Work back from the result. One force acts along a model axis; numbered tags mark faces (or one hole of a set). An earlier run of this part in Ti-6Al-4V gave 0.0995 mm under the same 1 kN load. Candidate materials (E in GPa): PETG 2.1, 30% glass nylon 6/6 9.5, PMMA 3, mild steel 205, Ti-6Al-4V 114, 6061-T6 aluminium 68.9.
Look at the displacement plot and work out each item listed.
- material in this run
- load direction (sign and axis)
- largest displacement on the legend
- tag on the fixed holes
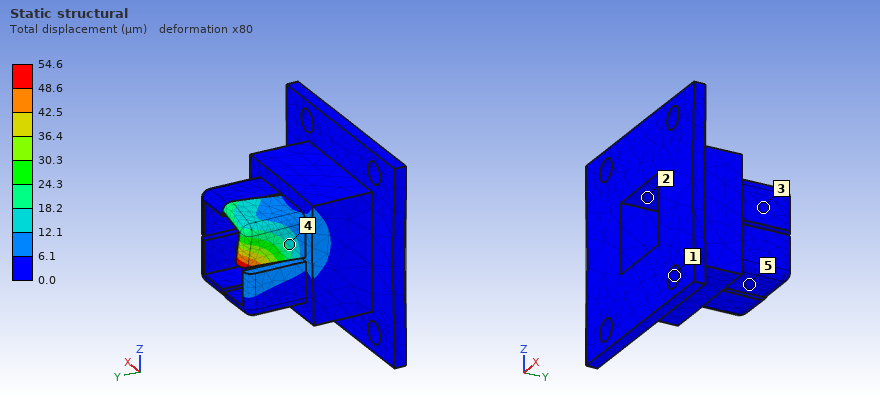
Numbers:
mild steel
+X
54.6 µm
1
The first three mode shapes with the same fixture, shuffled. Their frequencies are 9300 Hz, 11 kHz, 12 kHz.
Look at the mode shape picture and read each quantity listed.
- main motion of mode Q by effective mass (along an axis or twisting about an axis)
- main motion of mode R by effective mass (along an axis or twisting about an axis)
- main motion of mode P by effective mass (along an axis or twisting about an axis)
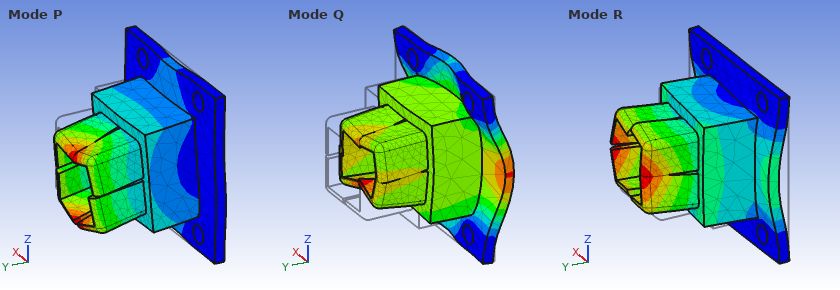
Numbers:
along Y
along X
along Z
